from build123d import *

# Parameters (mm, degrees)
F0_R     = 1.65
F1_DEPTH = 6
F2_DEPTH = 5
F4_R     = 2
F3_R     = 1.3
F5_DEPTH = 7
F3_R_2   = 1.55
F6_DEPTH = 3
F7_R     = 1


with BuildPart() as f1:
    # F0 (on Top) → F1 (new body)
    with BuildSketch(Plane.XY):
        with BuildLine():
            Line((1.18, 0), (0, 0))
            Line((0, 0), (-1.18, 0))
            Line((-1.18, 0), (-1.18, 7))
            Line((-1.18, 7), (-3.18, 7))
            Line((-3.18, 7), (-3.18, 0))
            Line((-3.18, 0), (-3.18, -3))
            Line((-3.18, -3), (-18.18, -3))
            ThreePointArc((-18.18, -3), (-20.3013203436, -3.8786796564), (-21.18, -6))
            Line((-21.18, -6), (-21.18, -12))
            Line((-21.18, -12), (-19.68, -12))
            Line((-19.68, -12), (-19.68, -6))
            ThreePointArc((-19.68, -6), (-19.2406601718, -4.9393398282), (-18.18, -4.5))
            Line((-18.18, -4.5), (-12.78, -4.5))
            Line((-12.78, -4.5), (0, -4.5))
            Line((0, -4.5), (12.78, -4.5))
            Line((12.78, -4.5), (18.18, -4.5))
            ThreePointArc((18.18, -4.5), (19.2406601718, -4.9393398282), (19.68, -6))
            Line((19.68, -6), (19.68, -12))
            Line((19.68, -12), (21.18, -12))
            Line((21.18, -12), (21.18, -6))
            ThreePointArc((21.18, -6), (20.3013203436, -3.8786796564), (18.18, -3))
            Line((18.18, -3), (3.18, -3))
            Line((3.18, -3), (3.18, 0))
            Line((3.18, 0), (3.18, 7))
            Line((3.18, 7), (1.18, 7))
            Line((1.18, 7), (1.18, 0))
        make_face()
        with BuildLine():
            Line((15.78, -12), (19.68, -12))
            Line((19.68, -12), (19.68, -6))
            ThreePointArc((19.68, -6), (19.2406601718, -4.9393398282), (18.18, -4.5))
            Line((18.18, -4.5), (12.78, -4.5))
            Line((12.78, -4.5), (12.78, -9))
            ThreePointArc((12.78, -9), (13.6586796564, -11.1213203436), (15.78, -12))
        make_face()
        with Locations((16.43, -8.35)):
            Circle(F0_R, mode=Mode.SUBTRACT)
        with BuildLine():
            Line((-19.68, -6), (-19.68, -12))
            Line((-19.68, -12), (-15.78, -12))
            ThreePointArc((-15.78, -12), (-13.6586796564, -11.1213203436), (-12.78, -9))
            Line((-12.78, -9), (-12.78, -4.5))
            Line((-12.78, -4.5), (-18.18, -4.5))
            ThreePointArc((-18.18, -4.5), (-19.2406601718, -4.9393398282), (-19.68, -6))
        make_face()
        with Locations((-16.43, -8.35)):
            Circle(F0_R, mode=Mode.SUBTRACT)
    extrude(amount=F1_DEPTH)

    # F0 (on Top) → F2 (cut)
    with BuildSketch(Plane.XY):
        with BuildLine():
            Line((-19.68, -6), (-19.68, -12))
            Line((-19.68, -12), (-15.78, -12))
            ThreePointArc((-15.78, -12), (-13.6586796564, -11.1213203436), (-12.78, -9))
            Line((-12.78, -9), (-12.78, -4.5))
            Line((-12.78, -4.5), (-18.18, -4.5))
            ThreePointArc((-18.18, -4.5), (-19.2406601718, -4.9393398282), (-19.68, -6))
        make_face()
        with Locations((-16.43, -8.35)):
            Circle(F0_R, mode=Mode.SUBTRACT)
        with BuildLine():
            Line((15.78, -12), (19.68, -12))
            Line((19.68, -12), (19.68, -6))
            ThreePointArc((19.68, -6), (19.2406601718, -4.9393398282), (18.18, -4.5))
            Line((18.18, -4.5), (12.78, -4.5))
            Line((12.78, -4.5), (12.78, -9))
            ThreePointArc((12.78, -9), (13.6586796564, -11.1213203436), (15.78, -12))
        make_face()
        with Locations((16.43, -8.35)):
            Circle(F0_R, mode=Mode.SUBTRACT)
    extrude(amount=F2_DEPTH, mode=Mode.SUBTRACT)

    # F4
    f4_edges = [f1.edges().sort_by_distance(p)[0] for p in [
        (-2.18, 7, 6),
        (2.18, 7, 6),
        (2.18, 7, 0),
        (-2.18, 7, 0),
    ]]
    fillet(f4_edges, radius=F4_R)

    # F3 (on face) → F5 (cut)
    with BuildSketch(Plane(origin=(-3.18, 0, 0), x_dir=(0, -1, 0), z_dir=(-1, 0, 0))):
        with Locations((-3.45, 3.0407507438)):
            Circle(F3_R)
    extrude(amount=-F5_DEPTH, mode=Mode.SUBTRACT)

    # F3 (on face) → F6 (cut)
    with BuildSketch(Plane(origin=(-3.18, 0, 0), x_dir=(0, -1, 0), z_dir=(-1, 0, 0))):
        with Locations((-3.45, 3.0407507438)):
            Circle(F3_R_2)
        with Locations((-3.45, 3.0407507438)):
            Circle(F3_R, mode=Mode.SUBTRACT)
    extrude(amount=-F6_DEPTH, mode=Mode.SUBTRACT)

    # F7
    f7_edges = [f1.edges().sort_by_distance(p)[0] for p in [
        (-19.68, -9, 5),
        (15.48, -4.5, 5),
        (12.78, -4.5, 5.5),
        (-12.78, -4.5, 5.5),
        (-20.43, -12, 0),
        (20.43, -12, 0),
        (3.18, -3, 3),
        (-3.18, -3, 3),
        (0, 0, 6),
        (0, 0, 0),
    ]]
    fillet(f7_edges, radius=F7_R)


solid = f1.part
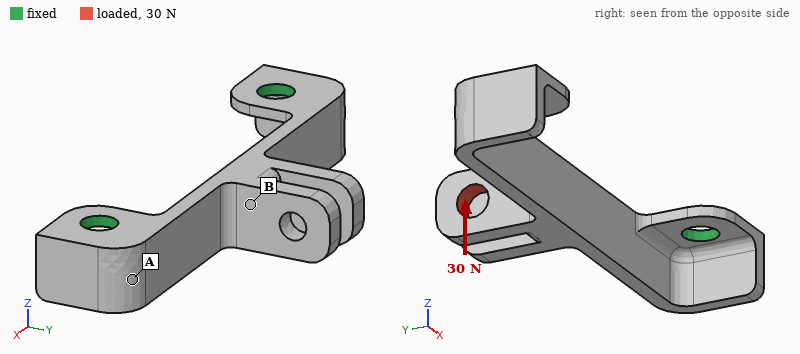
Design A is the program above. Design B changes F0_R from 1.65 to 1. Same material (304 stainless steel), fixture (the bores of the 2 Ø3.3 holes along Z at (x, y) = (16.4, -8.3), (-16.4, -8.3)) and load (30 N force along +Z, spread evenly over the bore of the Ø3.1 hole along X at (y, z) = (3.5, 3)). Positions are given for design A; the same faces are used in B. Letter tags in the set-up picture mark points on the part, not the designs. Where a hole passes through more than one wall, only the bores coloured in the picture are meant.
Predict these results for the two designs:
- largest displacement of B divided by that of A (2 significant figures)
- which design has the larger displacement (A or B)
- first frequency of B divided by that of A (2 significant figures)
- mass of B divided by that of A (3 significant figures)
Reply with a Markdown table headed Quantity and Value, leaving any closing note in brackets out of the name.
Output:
| Quantity | Value |
|---|---|
| largest displacement of B divided by that of A | 1.2 |
| which design has the larger displacement | B |
| first frequency of B divided by that of A | 0.90 |
| mass of B divided by that of A | 1.01 |
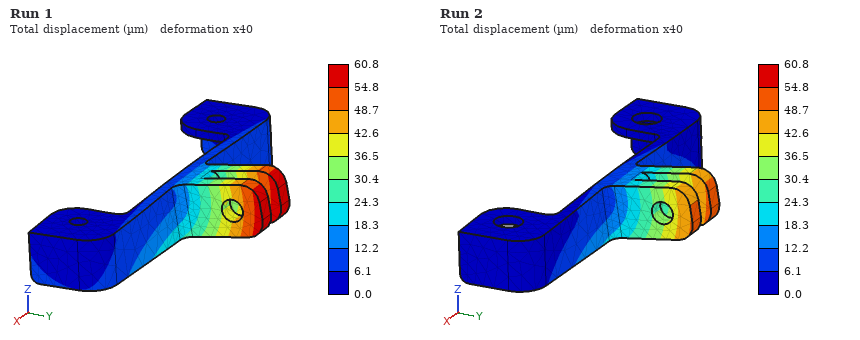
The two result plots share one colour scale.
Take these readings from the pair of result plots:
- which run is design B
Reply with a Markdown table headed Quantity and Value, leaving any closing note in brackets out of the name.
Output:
| Quantity | Value |
|---|---|
| which run is design B | Run 1 |
